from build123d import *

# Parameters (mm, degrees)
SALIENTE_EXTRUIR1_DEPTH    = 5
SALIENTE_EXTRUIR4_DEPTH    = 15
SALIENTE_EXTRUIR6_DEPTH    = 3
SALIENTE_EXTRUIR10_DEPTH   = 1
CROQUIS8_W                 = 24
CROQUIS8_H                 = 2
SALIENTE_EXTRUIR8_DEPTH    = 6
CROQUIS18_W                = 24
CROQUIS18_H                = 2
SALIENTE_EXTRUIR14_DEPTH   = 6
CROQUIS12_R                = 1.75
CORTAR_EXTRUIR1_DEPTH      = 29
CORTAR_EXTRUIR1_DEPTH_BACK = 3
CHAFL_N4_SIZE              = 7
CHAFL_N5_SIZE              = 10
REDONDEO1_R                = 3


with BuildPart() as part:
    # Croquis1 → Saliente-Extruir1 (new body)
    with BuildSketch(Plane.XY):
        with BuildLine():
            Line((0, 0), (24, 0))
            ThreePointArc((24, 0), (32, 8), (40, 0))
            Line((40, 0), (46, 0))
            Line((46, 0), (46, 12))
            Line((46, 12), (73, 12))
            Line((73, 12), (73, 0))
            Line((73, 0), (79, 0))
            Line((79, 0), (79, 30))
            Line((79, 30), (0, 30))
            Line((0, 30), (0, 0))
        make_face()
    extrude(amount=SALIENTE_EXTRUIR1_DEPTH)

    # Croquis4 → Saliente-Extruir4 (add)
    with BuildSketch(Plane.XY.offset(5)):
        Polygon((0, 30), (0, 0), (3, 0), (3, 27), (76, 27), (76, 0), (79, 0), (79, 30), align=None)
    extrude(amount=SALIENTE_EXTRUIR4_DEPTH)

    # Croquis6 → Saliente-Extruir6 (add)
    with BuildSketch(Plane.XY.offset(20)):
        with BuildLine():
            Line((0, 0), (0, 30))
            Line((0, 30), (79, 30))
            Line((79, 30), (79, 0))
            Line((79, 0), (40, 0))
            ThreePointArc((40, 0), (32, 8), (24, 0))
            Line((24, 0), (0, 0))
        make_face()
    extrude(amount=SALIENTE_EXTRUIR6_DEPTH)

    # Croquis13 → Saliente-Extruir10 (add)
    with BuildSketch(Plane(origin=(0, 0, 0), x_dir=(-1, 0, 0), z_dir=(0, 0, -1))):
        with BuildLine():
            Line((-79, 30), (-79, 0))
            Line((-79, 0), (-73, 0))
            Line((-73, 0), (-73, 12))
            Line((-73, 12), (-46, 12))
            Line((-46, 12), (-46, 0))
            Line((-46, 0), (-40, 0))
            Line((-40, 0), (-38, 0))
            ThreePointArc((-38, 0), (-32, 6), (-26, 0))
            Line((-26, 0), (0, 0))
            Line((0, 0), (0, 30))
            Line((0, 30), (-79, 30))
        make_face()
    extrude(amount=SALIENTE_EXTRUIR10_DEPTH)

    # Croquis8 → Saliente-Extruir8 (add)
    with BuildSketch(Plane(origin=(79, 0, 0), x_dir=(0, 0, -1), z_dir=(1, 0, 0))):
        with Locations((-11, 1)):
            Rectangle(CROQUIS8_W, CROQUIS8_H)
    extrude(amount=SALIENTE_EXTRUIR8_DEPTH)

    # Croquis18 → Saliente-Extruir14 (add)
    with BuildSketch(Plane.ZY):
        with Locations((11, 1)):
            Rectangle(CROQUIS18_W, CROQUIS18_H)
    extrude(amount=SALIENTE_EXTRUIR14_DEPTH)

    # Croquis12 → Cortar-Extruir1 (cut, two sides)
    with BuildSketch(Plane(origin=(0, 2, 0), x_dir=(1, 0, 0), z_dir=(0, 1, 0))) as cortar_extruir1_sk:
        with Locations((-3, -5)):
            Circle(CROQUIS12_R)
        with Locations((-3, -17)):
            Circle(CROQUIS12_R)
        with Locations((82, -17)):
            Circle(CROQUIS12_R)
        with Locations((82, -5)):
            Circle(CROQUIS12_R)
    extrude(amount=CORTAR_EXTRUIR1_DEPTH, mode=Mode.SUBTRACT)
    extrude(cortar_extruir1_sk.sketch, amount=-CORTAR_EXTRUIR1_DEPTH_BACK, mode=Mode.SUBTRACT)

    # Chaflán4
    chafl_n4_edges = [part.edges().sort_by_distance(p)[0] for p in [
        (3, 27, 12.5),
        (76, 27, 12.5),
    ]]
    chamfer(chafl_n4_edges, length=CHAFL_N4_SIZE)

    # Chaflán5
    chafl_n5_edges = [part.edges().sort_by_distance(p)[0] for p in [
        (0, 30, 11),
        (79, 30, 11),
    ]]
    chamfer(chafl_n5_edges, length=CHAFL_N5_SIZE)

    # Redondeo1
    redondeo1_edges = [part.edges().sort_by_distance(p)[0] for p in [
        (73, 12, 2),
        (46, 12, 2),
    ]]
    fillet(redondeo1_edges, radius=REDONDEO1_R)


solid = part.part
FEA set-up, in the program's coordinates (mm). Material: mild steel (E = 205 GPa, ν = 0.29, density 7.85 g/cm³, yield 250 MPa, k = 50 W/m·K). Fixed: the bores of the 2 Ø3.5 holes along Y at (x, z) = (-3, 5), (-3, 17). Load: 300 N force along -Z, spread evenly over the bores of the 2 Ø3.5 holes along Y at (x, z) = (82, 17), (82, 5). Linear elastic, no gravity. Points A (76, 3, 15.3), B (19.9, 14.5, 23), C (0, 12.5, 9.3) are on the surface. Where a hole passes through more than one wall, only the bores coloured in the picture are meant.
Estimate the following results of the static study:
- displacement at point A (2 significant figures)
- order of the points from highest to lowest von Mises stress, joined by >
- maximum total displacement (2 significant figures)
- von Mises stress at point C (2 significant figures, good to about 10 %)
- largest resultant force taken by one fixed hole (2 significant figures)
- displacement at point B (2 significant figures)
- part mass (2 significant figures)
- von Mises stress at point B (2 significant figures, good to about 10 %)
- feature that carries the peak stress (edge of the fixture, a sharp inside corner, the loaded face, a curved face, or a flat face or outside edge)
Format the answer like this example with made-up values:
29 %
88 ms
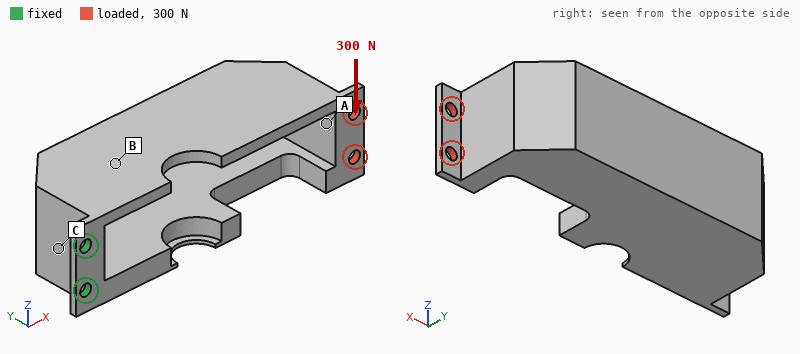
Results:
0.34 mm
C > B > A
0.39 mm
71 MPa
1.5 kN
0.067 mm
180 g
38 MPa
edge of the fixture
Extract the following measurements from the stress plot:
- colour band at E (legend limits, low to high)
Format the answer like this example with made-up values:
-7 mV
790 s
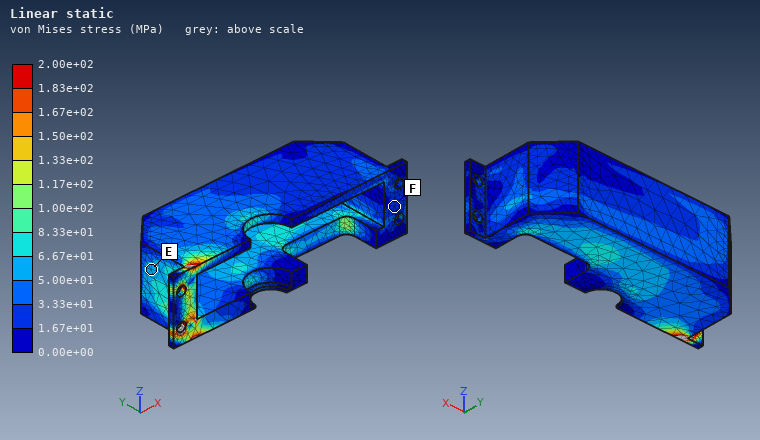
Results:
5.00e+01 to 6.67e+01 MPa
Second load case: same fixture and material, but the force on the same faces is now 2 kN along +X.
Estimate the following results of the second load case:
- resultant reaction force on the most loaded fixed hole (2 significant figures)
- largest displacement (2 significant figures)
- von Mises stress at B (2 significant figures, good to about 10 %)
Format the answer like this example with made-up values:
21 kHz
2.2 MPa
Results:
1.1 kN
0.14 mm
20 MPa
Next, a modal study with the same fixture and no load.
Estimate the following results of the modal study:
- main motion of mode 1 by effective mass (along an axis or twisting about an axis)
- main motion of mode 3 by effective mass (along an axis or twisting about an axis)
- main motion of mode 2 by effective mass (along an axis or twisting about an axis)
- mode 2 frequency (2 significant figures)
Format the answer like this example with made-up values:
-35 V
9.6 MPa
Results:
along Y
along Z
along Z
730 Hz
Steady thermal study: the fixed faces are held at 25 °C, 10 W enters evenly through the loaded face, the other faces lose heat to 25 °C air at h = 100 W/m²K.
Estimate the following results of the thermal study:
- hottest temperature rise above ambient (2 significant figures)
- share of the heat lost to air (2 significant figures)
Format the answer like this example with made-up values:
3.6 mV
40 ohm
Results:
58 K
96 %
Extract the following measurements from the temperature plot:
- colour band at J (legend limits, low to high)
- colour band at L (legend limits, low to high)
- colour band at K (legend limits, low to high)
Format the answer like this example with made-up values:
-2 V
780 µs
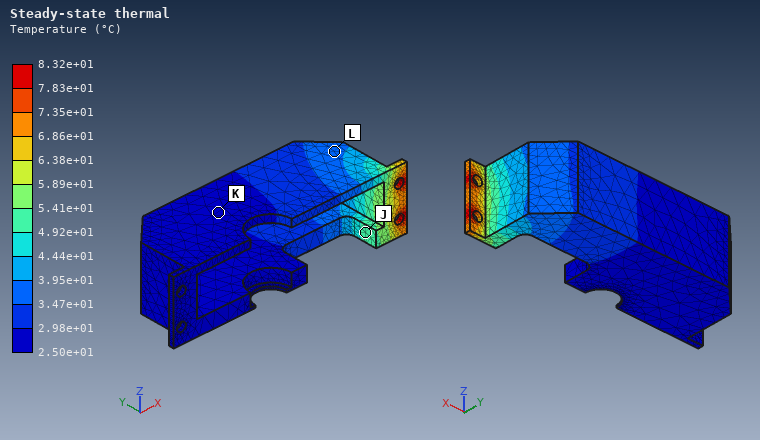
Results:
4.92e+01 to 5.41e+01 °C
3.47e+01 to 3.95e+01 °C
2.50e+01 to 2.98e+01 °C
